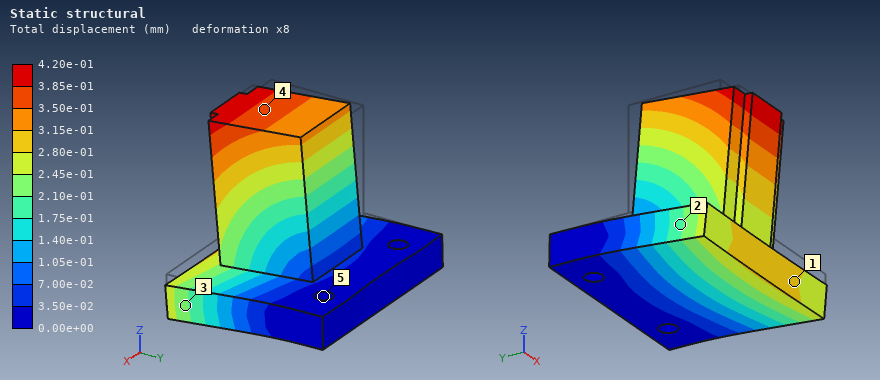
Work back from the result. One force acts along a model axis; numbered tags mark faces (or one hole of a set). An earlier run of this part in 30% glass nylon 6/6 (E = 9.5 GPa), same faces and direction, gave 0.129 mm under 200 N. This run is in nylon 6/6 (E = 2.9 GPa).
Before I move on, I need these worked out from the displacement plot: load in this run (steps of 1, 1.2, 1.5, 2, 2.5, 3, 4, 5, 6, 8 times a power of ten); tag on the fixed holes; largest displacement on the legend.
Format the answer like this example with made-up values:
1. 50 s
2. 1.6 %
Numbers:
1. 200 N
2. 5
3. 4.20e-01 mm
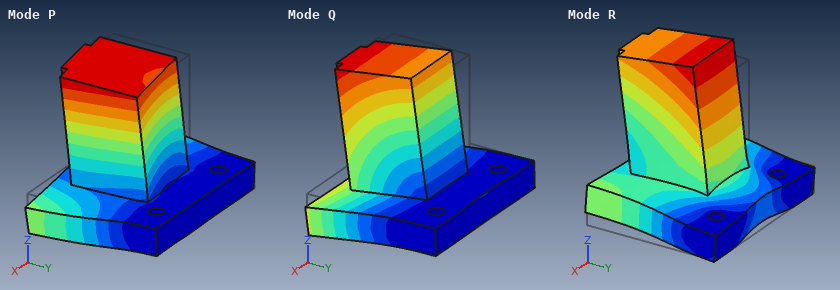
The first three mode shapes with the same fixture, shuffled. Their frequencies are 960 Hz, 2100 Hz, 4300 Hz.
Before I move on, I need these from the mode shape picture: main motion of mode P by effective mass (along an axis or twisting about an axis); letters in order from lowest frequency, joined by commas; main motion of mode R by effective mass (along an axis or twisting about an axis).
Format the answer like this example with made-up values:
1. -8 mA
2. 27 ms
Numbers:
1. along X
2. Q, P, R
3. along Z
